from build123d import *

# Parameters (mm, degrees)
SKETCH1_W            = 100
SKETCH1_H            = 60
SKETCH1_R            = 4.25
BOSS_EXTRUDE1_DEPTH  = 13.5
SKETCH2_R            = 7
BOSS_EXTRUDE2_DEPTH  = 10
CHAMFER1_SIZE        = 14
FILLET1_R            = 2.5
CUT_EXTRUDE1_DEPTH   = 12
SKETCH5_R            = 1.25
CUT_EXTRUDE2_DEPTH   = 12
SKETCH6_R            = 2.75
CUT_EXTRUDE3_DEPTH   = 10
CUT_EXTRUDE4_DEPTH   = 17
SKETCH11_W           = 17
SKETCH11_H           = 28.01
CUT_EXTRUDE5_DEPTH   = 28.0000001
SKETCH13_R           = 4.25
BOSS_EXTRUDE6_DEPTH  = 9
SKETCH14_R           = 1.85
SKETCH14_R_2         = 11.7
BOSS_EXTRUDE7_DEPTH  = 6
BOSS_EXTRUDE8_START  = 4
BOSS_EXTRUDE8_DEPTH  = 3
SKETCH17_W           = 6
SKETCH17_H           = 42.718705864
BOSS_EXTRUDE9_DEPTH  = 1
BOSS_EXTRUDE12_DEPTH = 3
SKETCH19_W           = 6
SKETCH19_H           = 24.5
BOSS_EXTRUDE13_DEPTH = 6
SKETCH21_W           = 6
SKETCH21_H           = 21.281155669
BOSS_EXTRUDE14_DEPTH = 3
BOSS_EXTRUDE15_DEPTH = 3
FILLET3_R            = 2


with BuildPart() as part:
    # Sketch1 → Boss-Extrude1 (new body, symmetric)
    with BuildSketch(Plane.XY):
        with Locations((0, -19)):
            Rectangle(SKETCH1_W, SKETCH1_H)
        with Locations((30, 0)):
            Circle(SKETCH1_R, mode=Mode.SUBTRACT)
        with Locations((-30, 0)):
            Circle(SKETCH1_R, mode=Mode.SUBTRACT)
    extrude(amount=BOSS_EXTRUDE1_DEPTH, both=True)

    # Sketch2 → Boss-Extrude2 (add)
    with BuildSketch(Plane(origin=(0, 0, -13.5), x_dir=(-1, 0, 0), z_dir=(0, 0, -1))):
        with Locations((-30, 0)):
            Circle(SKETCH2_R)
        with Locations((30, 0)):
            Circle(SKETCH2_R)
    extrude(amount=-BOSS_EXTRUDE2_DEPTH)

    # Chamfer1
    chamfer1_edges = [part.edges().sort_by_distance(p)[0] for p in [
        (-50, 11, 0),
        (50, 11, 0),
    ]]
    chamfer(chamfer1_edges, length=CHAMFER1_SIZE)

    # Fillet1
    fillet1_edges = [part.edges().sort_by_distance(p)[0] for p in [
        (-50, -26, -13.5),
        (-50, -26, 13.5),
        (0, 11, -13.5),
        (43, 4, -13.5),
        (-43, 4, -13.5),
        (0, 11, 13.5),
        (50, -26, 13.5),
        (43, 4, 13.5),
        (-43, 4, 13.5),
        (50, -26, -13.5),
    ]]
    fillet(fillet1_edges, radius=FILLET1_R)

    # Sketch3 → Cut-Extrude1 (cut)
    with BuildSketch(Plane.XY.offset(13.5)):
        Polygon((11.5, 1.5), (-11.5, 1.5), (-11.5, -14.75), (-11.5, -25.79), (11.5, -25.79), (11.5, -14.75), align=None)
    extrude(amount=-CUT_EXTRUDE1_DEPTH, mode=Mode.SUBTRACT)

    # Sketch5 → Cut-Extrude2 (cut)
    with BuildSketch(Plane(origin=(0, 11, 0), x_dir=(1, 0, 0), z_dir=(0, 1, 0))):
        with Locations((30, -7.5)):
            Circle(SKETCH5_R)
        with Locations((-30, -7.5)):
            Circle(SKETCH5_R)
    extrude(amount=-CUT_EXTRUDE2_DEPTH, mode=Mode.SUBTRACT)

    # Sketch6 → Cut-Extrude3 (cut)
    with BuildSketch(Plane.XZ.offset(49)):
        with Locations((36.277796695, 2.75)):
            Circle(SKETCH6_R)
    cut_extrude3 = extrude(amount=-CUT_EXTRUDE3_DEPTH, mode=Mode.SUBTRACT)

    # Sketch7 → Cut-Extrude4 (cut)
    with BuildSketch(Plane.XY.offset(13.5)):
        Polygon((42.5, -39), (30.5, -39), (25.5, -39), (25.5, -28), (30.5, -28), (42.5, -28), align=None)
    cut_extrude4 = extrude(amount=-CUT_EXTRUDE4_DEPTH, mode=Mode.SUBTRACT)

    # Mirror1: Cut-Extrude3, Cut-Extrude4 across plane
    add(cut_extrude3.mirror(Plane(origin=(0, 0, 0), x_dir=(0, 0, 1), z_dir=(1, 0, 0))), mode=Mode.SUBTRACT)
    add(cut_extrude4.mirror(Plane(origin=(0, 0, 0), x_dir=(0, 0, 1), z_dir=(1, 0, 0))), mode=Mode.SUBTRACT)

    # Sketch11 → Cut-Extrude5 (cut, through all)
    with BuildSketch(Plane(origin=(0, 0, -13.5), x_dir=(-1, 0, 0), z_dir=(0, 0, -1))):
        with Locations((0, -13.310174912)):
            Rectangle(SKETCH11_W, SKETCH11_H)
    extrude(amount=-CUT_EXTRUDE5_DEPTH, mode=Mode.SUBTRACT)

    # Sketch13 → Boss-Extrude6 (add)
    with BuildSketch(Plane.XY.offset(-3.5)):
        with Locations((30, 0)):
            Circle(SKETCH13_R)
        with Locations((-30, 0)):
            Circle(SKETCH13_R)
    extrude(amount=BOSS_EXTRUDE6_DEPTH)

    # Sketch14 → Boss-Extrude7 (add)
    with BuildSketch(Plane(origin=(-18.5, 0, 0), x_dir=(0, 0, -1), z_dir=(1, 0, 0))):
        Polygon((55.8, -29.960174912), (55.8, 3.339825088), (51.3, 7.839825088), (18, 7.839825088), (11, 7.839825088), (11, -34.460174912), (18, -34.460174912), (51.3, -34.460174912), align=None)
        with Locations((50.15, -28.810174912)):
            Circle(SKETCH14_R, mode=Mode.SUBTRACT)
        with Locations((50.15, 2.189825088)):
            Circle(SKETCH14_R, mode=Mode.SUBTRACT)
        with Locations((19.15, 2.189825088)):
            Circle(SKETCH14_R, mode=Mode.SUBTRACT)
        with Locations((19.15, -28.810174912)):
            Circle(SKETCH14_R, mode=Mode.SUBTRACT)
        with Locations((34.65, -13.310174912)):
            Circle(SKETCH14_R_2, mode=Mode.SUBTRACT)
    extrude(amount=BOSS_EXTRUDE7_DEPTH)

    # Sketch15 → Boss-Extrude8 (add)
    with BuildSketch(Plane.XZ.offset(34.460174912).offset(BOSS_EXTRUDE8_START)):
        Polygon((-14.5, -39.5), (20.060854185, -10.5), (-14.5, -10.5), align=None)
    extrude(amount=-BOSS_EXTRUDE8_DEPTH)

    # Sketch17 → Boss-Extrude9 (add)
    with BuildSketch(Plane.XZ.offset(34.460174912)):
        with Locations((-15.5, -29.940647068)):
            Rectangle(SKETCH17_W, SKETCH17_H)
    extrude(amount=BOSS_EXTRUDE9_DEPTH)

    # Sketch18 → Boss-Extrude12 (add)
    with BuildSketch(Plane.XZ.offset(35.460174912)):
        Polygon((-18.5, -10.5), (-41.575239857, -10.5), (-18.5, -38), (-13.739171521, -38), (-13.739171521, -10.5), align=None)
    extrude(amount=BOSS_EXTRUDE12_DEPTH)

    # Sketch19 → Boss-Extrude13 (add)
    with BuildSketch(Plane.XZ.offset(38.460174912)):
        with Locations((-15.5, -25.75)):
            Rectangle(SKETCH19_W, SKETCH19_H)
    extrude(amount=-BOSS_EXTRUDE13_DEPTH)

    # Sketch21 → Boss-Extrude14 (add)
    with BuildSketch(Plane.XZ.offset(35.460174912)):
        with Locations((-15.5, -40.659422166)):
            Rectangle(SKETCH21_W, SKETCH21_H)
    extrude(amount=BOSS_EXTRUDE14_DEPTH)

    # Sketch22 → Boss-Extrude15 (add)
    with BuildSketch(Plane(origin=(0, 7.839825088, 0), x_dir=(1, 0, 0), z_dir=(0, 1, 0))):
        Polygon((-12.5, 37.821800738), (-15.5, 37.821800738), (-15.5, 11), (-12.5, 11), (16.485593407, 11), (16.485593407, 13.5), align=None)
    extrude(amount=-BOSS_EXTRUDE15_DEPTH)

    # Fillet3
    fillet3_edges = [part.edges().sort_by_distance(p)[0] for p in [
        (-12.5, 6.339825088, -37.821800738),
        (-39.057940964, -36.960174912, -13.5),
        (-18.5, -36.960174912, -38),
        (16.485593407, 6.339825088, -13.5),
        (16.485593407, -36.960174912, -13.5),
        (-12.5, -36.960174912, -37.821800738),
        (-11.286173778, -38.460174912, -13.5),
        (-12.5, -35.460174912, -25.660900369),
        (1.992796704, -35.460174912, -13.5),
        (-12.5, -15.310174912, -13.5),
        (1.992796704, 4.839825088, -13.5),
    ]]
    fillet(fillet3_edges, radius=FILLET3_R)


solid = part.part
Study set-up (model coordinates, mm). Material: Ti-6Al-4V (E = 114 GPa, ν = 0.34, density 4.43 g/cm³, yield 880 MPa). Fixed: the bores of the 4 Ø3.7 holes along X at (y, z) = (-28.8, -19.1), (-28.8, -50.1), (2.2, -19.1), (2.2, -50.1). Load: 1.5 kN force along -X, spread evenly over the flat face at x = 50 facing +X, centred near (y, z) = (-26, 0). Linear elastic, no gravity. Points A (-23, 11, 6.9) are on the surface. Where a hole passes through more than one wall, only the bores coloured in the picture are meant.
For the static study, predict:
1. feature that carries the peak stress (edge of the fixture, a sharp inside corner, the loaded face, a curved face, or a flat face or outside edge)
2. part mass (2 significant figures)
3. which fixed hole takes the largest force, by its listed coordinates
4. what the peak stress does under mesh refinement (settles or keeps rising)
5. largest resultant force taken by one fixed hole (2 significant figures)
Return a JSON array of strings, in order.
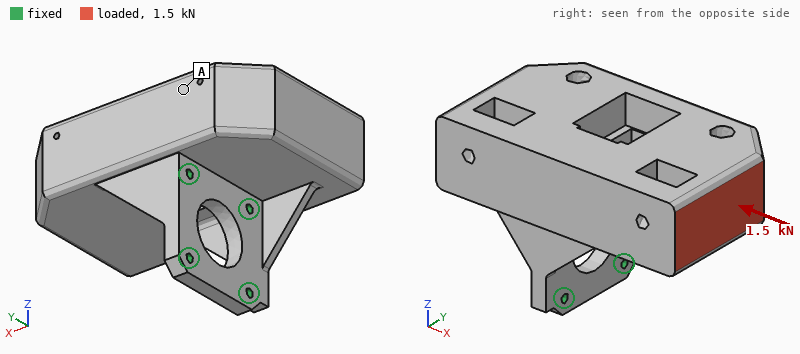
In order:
["edge of the fixture", "640 g", "(-28.8, -19.1)", "keeps rising", "1.6 kN"]
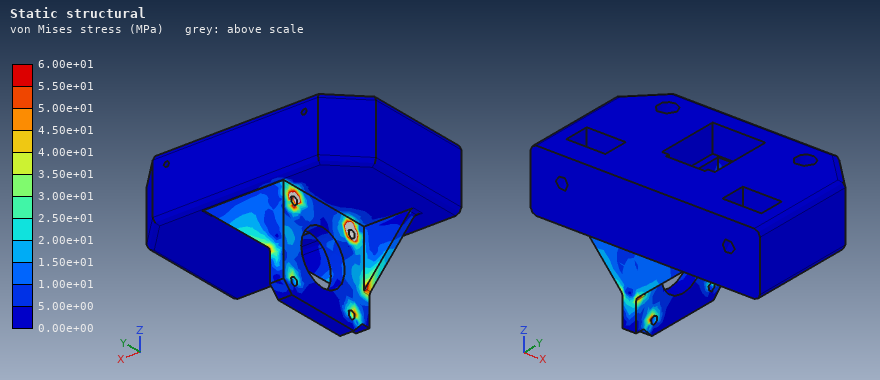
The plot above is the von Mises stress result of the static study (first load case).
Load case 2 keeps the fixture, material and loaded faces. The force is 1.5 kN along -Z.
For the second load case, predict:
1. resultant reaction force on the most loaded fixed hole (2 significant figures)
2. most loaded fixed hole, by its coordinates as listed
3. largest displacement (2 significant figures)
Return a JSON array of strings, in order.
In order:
["1.8 kN", "(-28.8, -19.1)", "0.20 mm"]
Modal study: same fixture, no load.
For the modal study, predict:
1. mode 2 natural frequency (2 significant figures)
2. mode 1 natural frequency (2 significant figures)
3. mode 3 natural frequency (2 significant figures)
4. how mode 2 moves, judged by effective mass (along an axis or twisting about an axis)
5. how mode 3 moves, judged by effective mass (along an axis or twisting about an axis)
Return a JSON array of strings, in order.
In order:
["2200 Hz", "1000 Hz", "4900 Hz", "along Y", "along Y"]
